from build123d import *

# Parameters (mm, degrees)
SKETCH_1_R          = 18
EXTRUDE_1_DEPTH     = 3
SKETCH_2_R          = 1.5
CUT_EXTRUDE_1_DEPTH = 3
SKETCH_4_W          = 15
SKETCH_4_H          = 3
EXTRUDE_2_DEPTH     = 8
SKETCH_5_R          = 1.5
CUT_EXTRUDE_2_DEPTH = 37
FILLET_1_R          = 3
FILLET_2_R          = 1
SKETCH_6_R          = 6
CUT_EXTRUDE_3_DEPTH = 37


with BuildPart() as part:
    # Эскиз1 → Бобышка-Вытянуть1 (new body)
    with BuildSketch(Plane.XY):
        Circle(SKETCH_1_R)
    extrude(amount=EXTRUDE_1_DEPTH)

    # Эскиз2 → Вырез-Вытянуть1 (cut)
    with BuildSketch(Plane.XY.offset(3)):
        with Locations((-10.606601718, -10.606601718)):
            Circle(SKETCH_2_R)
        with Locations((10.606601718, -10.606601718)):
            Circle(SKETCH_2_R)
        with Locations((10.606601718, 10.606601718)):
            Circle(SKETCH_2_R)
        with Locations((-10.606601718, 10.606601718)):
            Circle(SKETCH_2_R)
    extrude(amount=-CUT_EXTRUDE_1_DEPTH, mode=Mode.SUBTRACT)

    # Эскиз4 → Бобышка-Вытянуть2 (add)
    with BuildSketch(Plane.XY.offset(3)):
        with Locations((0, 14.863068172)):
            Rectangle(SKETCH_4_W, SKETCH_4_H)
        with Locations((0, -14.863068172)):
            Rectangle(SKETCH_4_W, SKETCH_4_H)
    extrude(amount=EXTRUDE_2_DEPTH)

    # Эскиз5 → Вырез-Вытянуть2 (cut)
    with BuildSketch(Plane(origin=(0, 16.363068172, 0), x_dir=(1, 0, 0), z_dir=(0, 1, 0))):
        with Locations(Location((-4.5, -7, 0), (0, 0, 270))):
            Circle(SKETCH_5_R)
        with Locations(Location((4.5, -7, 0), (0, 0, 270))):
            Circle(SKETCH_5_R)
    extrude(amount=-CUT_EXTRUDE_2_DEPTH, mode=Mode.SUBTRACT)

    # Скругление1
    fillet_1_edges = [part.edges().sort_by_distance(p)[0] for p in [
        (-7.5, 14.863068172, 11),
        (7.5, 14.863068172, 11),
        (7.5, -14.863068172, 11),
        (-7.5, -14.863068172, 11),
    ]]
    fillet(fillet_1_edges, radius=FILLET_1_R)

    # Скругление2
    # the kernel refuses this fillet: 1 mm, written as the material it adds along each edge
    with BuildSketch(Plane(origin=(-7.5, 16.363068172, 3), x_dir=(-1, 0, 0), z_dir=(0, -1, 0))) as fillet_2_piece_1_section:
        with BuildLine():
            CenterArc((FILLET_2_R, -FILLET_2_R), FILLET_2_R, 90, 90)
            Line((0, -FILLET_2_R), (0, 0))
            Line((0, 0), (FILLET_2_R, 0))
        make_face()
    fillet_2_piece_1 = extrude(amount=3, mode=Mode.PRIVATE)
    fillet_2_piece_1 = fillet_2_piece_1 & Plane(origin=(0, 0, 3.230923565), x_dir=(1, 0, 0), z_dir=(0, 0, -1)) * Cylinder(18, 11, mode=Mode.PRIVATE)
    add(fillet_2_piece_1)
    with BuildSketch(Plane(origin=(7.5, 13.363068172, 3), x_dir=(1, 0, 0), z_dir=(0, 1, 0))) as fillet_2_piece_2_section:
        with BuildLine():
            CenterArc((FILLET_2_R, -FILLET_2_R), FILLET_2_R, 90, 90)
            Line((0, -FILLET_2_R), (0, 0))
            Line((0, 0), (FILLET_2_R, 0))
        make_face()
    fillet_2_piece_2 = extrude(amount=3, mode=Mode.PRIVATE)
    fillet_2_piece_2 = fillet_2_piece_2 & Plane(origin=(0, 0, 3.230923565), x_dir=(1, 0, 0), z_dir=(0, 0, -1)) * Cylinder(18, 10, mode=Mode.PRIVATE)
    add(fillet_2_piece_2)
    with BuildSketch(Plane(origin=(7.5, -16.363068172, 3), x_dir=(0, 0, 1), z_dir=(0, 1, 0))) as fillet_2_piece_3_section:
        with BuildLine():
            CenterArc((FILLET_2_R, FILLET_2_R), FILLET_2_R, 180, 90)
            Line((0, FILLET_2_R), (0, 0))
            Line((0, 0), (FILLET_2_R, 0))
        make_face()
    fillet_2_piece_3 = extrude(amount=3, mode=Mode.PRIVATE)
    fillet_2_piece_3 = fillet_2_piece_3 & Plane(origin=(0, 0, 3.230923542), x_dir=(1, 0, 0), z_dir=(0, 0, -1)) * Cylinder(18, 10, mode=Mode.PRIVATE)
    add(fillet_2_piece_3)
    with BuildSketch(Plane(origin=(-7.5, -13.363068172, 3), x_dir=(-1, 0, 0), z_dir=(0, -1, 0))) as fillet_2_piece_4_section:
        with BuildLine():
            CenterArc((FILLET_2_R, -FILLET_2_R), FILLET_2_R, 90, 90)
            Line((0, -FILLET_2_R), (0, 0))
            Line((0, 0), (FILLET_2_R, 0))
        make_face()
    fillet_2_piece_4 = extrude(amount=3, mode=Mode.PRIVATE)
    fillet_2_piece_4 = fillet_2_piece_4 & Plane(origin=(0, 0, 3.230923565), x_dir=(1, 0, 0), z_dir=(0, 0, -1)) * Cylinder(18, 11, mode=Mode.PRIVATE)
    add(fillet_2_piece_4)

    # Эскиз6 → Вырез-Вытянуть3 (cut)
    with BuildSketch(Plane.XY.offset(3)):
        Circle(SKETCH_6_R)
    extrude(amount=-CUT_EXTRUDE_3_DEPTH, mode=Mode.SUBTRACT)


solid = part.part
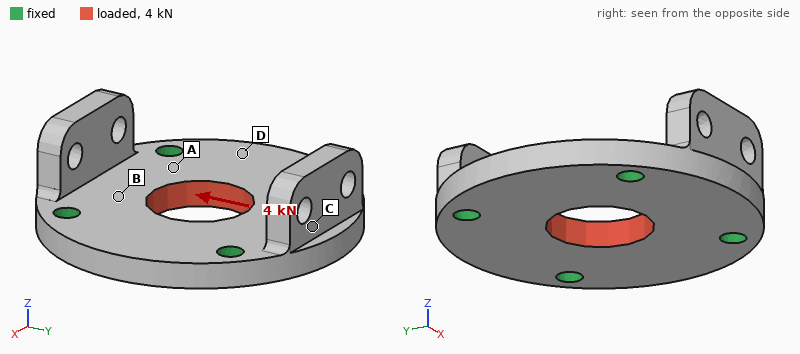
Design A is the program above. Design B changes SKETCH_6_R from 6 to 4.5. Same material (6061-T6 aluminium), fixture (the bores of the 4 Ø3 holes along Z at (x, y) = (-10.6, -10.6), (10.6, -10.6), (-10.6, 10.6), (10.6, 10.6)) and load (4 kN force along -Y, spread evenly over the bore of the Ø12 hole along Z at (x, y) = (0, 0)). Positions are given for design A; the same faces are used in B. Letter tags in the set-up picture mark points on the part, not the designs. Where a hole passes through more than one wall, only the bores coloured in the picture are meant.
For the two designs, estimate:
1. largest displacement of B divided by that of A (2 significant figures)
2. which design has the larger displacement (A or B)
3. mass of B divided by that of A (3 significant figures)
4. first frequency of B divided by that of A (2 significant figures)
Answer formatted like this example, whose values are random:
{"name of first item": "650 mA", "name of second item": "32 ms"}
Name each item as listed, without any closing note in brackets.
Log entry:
{"largest displacement of B divided by that of A": "1.1", "which design has the larger displacement": "B", "mass of B divided by that of A": "1.05", "first frequency of B divided by that of A": "1.0"}
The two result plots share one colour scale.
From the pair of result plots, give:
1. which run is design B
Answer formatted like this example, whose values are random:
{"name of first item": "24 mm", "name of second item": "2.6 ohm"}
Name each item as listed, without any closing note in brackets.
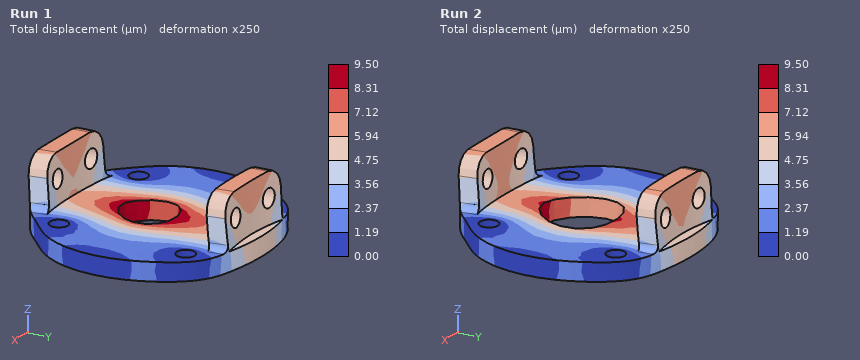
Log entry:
{"which run is design B": "Run 1"}
